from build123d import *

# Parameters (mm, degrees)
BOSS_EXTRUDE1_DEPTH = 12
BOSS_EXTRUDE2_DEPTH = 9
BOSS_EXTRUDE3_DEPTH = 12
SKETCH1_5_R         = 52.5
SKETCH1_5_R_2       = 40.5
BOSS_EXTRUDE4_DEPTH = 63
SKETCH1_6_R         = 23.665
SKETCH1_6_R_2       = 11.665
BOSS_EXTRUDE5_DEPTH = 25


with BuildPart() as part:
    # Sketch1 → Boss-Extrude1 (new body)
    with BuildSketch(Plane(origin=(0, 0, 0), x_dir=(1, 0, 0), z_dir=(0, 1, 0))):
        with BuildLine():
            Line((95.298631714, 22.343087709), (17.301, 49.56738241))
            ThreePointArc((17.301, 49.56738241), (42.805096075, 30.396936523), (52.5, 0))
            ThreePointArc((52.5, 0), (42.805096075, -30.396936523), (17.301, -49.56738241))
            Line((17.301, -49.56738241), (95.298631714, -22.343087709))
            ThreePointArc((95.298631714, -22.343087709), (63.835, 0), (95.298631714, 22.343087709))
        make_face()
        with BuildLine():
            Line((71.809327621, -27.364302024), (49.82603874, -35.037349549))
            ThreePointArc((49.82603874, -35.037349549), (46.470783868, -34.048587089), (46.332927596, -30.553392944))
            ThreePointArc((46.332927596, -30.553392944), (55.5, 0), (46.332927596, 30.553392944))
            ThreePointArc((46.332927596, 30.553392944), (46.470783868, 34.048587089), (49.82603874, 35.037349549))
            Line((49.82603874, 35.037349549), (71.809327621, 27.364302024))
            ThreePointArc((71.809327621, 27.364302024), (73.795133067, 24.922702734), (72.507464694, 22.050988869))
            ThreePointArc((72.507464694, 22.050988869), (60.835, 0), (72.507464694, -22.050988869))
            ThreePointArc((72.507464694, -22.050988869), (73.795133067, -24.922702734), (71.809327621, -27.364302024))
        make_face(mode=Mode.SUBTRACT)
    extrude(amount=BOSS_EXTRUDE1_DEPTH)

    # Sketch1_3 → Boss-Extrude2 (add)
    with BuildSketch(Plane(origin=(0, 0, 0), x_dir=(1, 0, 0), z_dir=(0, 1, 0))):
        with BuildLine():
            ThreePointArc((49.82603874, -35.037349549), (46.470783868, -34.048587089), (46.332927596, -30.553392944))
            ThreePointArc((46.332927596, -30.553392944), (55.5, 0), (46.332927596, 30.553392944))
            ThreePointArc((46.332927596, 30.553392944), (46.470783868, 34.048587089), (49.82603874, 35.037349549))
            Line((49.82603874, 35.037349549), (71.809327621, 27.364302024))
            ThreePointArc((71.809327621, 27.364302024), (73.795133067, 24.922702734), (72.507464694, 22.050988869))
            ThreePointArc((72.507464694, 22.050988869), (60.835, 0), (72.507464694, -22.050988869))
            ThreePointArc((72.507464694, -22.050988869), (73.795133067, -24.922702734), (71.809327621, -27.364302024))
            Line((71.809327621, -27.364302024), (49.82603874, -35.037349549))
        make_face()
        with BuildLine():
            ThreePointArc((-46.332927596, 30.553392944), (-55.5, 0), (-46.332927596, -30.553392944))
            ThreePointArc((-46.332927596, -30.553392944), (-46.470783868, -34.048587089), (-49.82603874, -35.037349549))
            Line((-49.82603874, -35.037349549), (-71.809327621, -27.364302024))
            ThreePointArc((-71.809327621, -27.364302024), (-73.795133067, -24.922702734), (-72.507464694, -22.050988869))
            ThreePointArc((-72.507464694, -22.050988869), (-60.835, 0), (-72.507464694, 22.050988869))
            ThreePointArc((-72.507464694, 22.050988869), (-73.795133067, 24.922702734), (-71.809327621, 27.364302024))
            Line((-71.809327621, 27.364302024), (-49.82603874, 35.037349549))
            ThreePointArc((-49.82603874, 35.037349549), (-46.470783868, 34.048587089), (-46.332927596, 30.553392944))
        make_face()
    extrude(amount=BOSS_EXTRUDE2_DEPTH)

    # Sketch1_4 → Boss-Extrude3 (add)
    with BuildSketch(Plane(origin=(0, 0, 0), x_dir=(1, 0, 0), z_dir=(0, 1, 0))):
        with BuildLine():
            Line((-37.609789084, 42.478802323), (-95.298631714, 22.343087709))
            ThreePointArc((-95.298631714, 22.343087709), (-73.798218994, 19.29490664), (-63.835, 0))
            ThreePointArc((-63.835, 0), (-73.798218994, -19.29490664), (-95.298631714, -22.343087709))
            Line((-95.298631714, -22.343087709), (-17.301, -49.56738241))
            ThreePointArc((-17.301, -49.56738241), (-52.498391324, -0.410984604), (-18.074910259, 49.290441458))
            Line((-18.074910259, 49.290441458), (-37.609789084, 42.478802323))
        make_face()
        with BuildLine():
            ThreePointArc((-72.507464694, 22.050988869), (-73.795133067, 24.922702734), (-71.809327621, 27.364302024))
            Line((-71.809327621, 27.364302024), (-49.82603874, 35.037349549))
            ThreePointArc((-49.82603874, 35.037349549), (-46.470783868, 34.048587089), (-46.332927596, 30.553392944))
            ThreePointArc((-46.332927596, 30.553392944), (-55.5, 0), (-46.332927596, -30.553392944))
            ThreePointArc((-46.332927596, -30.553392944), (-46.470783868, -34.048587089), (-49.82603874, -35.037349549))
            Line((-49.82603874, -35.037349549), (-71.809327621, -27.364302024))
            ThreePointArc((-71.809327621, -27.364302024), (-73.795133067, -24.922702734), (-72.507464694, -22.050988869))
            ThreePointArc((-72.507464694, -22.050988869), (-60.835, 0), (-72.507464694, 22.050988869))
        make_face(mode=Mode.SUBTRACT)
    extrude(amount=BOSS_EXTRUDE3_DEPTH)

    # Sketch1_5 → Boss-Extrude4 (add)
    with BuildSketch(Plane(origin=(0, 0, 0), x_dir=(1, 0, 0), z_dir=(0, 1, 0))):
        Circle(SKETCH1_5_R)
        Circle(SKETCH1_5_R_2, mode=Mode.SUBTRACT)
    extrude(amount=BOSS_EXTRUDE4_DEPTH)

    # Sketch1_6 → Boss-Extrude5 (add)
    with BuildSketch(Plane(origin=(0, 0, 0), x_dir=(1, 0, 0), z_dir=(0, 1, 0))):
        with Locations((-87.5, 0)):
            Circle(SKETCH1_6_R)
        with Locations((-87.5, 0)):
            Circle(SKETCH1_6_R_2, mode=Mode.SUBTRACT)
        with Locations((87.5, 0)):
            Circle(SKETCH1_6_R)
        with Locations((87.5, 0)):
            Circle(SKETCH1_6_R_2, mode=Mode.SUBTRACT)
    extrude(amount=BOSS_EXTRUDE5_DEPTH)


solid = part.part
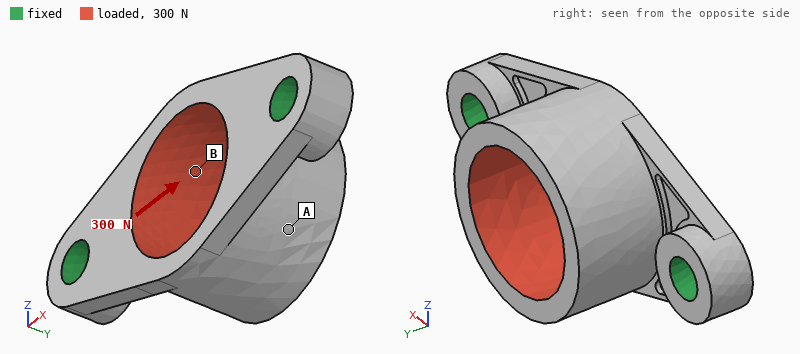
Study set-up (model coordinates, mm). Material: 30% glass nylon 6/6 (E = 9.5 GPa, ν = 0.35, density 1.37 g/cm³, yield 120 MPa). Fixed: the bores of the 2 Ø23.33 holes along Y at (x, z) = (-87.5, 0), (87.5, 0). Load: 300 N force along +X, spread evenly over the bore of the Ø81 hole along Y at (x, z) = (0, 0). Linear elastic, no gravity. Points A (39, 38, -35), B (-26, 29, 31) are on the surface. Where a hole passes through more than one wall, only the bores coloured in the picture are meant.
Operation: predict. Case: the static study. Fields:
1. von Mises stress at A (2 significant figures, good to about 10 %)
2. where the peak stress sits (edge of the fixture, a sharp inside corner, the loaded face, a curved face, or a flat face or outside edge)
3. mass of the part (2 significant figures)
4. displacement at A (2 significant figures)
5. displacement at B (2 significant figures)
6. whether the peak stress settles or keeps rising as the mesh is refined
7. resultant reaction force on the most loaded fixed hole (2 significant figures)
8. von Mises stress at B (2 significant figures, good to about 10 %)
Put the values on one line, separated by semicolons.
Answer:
0.076 MPa; edge of the fixture; 450 g; 4.4 µm; 3.5 µm; keeps rising; 160 N; 0.21 MPa
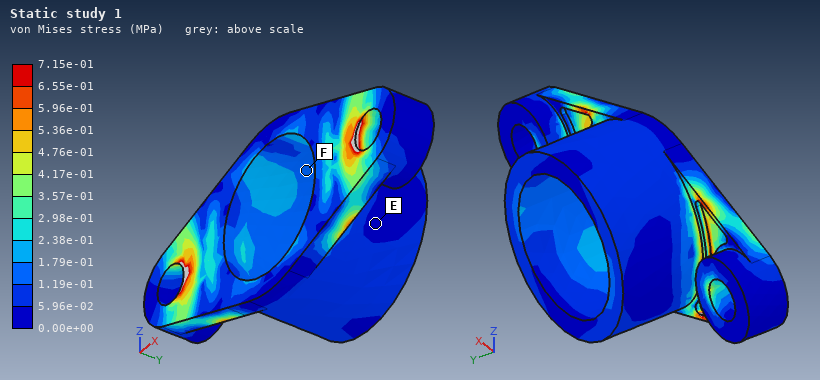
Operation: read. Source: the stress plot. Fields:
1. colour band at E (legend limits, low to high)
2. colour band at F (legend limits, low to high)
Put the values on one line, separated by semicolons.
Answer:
0.00e+00 to 5.96e-02 MPa; 1.19e-01 to 1.79e-01 MPa
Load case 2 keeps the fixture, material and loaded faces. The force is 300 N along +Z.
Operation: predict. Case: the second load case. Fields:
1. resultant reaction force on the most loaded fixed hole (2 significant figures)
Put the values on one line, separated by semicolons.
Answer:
150 N
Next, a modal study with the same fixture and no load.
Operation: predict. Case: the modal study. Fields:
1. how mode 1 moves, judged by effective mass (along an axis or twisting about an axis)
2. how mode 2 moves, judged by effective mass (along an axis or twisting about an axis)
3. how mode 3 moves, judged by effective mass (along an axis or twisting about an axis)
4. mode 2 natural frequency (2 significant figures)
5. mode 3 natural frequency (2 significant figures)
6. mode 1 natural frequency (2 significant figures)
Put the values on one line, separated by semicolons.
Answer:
along Z; along Y; along X; 1400 Hz; 2100 Hz; 640 Hz
